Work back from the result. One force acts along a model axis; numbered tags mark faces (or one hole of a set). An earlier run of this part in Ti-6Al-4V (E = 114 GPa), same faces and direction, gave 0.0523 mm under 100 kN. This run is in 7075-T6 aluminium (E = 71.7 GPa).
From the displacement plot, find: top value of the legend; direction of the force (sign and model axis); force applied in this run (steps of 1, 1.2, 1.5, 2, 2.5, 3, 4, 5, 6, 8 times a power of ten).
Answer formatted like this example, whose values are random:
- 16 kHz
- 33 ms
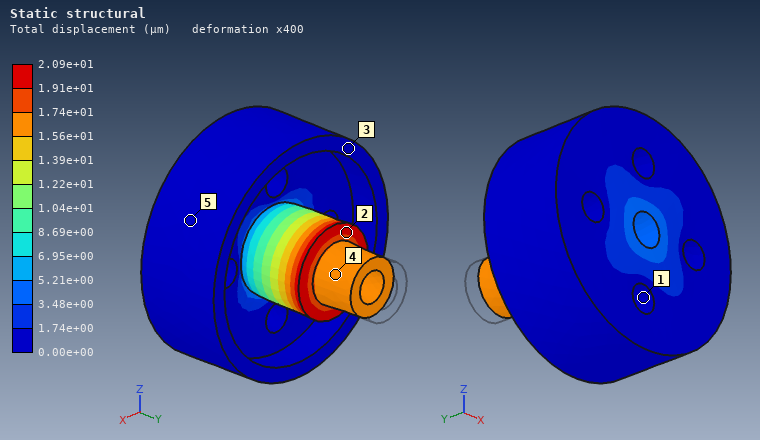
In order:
- 2.09e+01 µm
- -Y
- 25 kN
